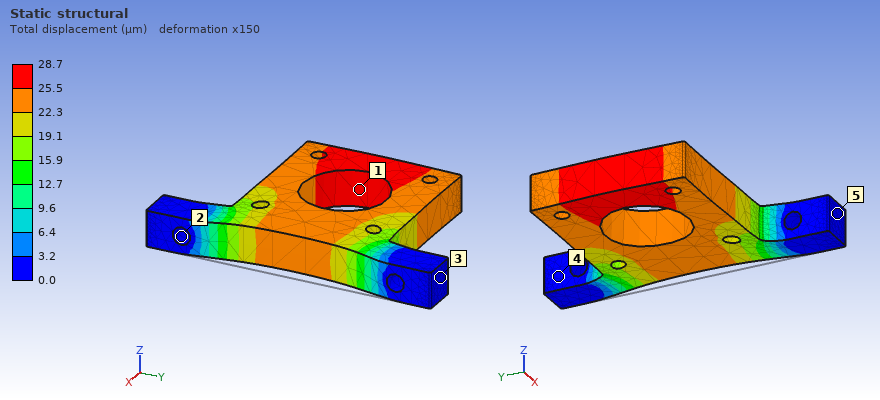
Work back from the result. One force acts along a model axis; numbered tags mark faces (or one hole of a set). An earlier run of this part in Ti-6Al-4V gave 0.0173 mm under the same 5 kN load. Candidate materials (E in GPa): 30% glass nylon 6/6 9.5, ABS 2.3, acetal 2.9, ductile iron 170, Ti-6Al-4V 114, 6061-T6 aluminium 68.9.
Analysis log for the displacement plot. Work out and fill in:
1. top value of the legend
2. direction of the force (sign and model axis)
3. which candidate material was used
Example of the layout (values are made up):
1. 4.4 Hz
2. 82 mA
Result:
1. 28.7 µm
2. -X
3. 6061-T6 aluminium
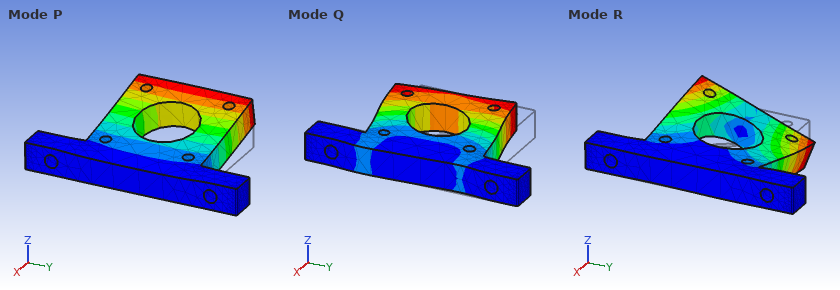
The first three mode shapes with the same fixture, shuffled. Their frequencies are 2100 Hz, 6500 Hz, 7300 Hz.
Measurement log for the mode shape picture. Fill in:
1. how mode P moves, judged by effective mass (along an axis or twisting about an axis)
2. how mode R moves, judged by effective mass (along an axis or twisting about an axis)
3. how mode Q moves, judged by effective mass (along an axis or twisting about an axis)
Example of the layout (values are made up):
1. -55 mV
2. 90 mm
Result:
1. along Z
2. twisting about X
3. along Y
